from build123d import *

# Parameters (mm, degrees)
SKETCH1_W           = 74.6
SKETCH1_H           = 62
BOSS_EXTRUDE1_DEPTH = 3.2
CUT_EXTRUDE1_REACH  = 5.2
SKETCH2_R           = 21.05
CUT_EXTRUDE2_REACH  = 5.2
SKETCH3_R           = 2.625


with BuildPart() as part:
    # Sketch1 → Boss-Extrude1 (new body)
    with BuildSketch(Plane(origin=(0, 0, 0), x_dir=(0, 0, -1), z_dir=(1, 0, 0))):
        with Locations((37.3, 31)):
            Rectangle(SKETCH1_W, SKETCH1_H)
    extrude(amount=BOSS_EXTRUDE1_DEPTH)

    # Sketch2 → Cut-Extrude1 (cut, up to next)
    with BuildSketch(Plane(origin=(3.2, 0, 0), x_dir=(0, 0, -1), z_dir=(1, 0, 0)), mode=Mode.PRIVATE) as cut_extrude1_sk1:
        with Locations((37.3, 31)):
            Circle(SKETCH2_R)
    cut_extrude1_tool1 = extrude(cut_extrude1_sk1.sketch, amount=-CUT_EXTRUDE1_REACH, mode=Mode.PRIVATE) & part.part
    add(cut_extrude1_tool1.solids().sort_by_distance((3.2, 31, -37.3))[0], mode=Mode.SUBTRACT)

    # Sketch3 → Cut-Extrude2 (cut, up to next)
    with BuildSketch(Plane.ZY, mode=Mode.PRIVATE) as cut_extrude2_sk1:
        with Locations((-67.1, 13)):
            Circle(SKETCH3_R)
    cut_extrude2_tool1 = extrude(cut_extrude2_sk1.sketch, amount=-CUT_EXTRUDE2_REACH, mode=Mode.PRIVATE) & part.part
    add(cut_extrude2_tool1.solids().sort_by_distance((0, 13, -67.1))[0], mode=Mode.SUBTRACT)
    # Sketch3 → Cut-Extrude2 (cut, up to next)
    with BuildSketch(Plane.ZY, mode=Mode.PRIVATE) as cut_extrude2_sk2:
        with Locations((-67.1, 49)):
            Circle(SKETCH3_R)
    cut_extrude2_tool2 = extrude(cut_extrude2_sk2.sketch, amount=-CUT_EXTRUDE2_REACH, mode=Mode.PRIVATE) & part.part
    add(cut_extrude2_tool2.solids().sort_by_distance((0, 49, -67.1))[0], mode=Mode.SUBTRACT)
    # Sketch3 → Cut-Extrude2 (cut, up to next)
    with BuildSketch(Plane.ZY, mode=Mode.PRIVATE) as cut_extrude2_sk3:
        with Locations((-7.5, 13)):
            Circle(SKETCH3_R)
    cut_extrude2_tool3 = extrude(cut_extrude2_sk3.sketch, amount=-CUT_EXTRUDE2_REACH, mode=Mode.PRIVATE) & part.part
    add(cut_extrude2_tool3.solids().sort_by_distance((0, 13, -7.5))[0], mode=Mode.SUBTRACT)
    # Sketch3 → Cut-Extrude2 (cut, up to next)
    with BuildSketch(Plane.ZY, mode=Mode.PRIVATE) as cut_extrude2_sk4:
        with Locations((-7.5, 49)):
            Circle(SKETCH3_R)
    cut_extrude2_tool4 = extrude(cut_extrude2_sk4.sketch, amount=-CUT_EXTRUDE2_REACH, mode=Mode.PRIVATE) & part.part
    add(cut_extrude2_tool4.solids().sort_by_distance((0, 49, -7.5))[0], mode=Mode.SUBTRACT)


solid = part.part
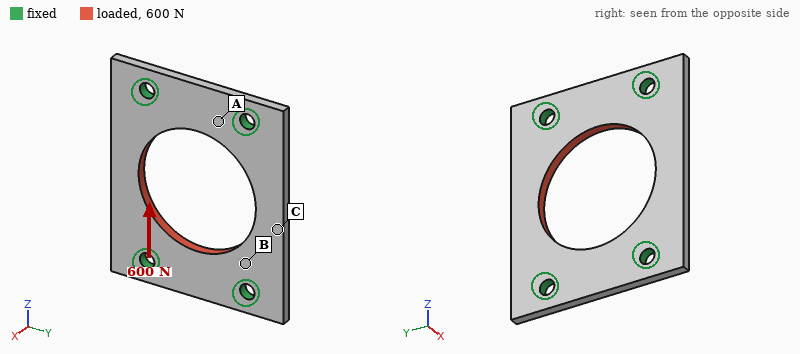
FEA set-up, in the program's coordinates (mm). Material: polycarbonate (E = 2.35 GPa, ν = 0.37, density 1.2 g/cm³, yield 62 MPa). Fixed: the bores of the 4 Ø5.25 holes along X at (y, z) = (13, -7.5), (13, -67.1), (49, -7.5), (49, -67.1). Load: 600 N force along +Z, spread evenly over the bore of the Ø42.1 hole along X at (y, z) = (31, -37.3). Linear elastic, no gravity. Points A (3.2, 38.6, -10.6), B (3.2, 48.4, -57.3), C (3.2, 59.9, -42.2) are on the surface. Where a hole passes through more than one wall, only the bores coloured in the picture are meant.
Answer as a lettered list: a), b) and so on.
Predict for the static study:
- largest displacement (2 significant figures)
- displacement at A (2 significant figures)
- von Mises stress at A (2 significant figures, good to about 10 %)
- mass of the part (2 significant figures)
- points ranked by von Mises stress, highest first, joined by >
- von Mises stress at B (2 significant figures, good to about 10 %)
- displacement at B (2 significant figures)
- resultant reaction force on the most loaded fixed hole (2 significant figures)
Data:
a) 25 µm
b) 17 µm
c) 1.6 MPa
d) 12 g
e) B > A > C
f) 2.8 MPa
g) 10 µm
h) 150 N
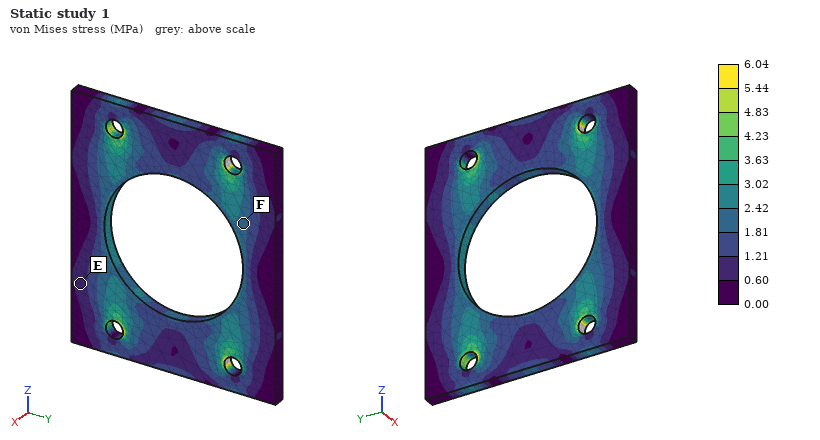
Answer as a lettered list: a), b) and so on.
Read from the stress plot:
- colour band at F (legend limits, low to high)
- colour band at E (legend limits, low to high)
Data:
a) 1.81 to 2.42 MPa
b) 0.60 to 1.21 MPa
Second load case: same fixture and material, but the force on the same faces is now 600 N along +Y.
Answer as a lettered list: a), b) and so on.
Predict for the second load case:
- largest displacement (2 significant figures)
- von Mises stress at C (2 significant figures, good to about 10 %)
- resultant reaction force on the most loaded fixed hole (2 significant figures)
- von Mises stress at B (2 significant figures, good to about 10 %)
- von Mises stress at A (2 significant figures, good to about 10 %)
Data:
a) 93 µm
b) 4.2 MPa
c) 150 N
d) 2.9 MPa
e) 3.5 MPa
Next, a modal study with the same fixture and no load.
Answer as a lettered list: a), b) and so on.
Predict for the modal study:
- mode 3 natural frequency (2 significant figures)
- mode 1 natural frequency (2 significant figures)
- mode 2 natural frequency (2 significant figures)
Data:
a) 3400 Hz
b) 1500 Hz
c) 1500 Hz
